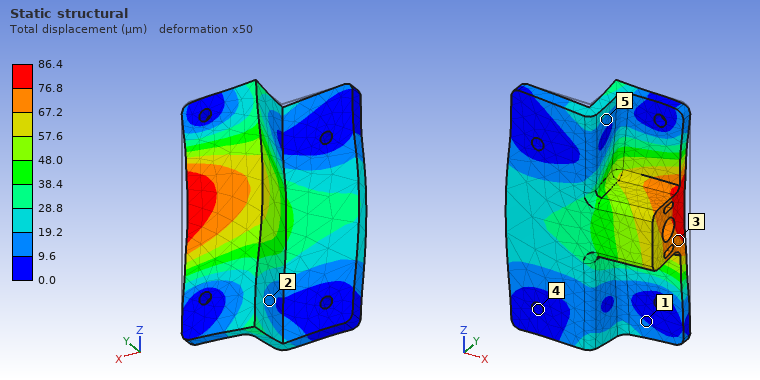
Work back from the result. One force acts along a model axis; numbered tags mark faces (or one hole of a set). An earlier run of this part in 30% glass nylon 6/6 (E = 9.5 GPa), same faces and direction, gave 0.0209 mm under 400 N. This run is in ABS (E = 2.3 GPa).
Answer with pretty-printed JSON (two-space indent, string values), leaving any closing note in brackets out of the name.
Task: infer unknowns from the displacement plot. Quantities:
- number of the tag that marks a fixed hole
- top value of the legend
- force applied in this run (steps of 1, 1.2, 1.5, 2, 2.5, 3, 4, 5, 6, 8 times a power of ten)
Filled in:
{
  "number of the tag that marks a fixed hole": "4",
  "top value of the legend": "86.4 µm",
  "force applied in this run": "400 N"
}
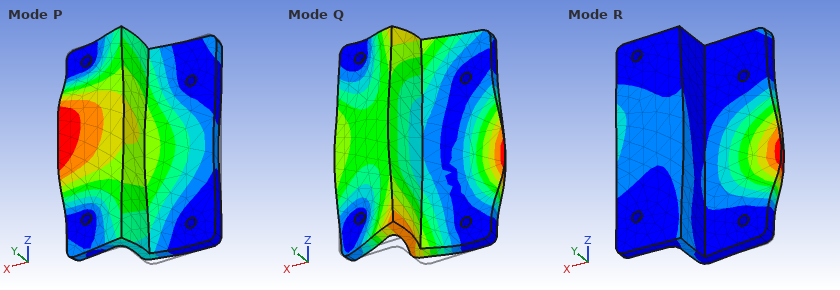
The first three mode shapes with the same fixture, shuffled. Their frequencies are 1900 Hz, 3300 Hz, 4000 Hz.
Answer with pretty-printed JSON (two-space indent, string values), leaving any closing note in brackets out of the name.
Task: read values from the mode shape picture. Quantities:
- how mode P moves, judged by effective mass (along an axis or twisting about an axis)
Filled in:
{
  "how mode P moves, judged by effective mass": "along Y"
}
